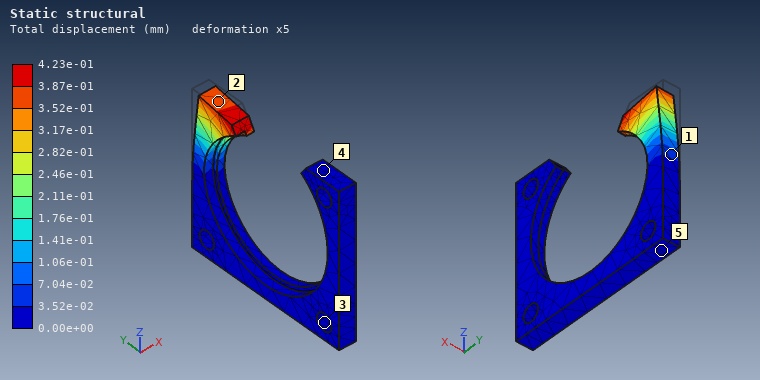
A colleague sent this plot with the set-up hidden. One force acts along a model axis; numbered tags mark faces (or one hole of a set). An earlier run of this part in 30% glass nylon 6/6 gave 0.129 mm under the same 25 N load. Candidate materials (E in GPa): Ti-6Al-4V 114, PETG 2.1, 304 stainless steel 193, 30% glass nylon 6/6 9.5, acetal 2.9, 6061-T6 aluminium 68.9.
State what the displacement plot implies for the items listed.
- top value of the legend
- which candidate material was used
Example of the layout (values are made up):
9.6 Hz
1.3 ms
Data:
4.23e-01 mm
acetal
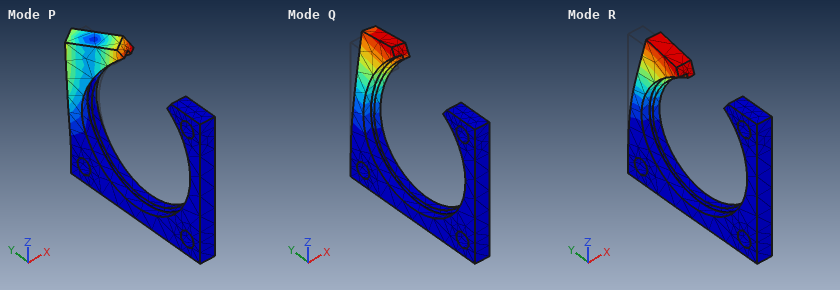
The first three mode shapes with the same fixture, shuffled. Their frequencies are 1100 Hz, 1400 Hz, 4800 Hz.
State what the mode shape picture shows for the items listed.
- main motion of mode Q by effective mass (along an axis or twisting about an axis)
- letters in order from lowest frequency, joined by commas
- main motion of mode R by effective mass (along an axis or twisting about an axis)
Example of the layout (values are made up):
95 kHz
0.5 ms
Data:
along X
Q, R, P
along Y
